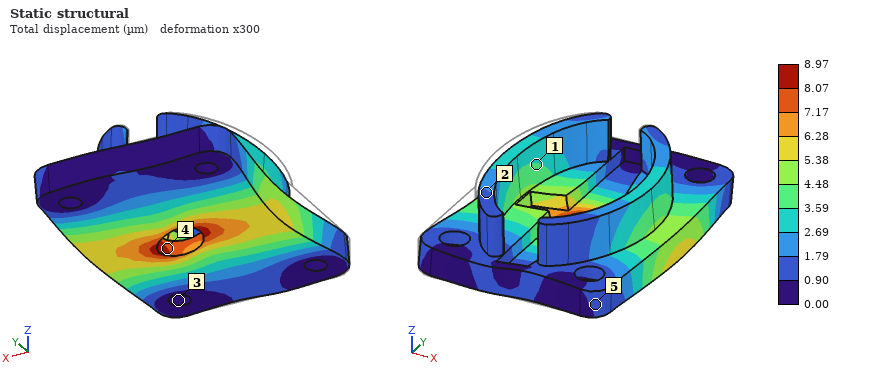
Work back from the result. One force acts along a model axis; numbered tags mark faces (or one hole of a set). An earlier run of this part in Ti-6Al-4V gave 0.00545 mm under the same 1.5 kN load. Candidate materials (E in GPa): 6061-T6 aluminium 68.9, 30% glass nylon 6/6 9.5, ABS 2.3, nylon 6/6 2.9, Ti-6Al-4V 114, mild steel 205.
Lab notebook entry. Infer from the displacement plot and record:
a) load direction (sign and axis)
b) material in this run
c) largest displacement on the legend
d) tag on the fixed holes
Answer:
+X
6061-T6 aluminium
8.97 µm
3
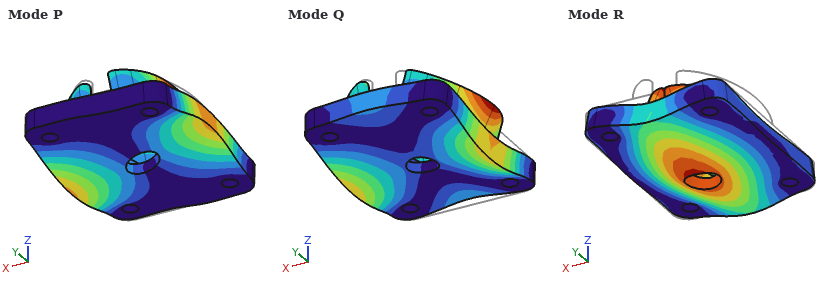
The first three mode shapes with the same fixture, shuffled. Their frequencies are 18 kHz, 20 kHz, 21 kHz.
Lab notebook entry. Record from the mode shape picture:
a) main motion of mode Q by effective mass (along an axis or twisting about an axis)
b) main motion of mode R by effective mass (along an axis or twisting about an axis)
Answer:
along Z
along Z
